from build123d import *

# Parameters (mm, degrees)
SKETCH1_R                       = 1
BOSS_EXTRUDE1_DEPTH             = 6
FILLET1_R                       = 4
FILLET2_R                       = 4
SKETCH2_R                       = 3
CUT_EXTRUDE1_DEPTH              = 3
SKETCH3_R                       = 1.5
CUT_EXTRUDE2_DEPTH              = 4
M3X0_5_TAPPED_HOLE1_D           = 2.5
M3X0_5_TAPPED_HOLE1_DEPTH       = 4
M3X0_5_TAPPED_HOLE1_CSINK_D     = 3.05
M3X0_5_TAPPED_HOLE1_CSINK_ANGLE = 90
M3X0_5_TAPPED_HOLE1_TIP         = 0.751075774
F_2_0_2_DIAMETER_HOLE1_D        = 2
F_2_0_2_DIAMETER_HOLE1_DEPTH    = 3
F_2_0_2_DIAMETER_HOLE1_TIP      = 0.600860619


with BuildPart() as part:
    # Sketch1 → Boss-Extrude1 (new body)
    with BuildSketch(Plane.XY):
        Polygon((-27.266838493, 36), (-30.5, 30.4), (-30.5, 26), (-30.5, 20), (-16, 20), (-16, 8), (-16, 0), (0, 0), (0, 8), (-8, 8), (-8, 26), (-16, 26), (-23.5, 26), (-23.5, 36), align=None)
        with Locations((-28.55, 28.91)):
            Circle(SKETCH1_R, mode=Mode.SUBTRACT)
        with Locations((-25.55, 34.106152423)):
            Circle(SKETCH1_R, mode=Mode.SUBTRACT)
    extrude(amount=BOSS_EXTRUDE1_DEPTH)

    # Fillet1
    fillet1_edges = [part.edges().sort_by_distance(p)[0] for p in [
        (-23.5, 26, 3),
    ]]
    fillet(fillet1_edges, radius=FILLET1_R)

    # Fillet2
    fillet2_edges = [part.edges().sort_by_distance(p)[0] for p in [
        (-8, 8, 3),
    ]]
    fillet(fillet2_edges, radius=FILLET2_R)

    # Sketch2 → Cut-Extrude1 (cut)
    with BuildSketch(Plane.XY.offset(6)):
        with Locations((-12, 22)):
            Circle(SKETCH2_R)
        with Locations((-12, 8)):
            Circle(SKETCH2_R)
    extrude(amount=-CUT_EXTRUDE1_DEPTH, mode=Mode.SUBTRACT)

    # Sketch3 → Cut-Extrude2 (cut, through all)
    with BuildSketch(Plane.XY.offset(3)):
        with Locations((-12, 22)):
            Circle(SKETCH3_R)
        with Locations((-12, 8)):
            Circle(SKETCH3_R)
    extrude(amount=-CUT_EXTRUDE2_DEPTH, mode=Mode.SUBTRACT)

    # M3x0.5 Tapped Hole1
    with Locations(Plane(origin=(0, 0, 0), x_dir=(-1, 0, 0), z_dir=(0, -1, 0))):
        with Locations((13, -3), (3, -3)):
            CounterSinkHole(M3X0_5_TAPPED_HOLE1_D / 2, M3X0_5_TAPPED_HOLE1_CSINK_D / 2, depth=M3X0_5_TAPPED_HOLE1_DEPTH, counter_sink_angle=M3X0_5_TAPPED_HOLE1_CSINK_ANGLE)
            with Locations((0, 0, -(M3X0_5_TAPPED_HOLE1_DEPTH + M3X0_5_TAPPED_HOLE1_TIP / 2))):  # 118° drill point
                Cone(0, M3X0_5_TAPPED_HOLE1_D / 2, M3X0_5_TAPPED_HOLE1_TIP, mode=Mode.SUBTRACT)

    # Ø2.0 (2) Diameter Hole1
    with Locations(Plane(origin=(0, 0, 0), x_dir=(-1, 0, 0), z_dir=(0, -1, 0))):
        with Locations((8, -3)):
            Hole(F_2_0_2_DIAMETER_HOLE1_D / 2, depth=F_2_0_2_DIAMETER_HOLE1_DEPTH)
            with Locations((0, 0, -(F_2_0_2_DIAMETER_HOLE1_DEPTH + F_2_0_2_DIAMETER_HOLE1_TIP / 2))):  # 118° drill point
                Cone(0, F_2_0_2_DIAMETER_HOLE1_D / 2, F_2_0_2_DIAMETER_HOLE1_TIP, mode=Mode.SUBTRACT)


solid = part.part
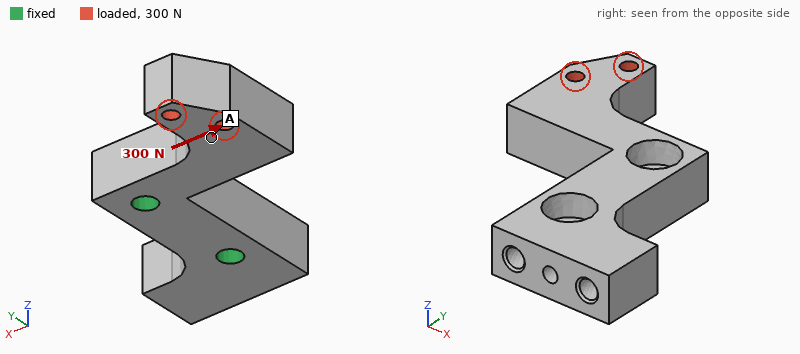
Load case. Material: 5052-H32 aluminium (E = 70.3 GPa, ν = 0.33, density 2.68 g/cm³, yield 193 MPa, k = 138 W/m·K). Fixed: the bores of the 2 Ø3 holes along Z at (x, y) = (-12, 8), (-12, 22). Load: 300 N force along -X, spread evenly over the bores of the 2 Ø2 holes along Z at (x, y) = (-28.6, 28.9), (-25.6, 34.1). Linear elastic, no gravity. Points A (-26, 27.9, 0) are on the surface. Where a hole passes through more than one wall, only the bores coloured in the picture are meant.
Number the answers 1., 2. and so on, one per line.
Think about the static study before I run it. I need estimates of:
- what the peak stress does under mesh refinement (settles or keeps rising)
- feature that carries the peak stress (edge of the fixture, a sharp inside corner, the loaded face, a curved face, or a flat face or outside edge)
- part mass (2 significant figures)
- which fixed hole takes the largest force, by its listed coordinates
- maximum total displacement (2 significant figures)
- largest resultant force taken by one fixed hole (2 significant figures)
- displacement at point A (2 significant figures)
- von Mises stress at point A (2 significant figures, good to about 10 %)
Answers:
1. keeps rising
2. edge of the fixture
3. 6.1 g
4. (-12, 22)
5. 83 µm
6. 410 N
7. 47 µm
8. 15 MPa
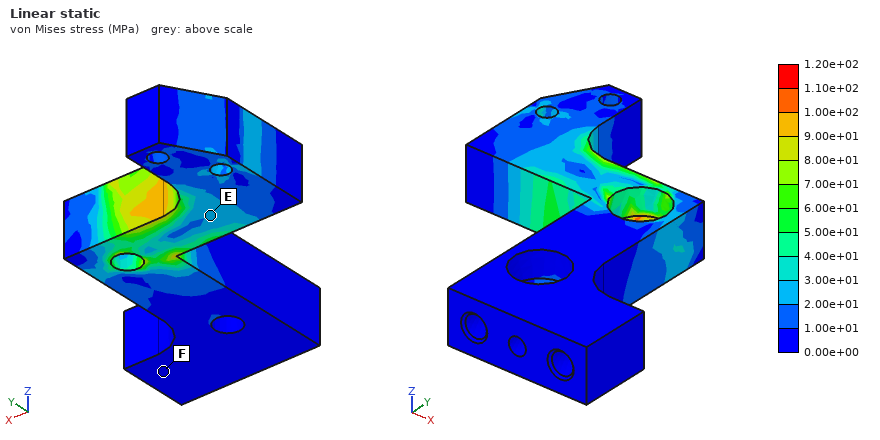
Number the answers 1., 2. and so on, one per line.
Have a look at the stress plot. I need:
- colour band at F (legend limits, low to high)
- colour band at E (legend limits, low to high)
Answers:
1. 0.00e+00 to 1.00e+01 MPa
2. 2.00e+01 to 3.00e+01 MPa
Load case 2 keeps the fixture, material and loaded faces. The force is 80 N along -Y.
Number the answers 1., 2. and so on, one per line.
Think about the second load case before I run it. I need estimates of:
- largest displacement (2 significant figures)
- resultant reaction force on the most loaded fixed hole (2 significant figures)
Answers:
1. 22 µm
2. 69 N
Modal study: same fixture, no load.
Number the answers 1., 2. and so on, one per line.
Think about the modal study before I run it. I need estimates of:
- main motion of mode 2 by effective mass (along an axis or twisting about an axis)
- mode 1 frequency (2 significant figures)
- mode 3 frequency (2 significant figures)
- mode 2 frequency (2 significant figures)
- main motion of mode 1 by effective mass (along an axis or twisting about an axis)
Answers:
1. along Y
2. 6600 Hz
3. 16 kHz
4. 8200 Hz
5. along Z
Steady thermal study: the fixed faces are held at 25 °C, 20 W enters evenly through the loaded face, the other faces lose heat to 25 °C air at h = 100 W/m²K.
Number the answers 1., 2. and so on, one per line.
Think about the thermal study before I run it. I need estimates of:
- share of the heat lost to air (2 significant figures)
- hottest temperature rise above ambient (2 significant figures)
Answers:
1. 15 %
2. 72 K
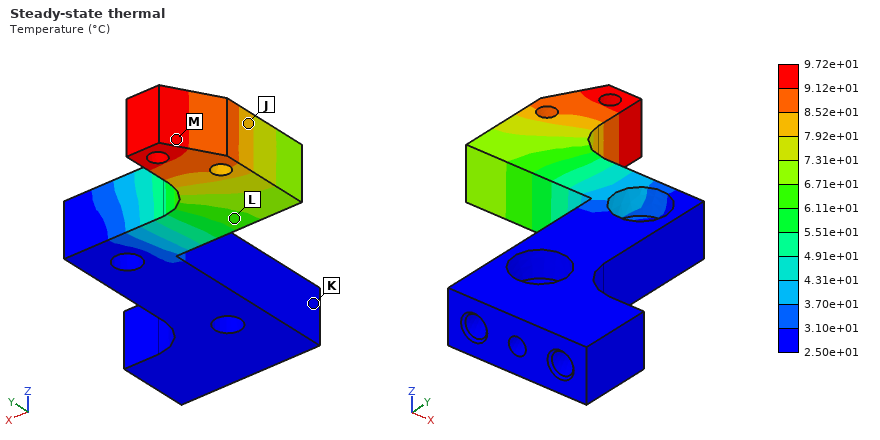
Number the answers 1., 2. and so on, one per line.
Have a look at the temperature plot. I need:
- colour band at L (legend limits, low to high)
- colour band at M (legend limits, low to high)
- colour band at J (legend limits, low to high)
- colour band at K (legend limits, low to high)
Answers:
1. 6.11e+01 to 6.71e+01 °C
2. 9.12e+01 to 9.72e+01 °C
3. 7.92e+01 to 8.52e+01 °C
4. 2.50e+01 to 3.10e+01 °C
